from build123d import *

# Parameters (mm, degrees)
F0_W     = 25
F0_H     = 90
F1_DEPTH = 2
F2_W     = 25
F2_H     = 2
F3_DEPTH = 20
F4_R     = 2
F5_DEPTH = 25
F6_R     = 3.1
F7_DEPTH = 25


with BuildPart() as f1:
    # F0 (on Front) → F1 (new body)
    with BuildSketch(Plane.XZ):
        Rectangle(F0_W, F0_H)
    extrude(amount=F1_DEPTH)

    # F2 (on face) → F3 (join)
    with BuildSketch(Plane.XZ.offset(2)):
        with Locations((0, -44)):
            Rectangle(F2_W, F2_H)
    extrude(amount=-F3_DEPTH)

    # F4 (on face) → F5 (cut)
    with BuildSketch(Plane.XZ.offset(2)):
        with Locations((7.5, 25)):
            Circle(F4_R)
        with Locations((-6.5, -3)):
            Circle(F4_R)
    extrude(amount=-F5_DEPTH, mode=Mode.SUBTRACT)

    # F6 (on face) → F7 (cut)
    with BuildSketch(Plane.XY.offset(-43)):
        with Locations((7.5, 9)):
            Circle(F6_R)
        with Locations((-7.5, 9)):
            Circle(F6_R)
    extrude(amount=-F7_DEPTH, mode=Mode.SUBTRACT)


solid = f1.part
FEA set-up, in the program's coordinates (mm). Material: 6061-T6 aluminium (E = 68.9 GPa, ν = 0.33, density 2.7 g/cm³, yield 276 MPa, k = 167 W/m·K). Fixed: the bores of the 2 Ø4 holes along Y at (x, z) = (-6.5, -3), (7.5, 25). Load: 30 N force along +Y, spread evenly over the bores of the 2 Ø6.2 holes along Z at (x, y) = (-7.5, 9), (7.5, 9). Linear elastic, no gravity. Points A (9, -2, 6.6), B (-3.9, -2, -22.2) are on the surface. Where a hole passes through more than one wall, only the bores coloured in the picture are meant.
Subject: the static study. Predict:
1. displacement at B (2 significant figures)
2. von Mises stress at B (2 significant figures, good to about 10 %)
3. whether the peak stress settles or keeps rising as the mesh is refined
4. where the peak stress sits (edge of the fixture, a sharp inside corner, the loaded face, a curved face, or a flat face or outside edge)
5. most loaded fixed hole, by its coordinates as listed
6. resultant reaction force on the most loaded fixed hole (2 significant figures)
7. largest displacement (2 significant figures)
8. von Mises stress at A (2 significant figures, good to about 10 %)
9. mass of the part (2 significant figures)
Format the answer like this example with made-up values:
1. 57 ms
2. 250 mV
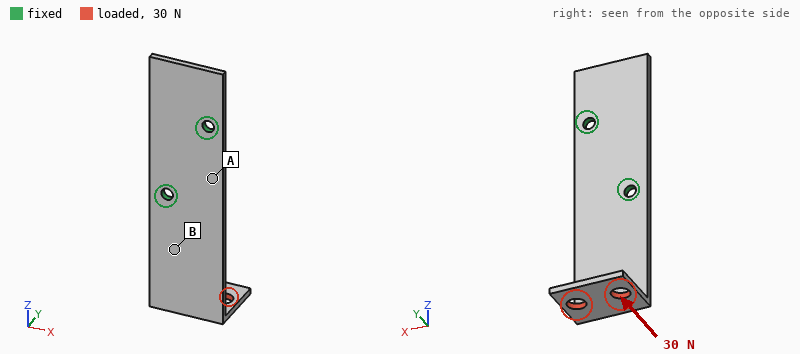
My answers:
1. 0.17 mm
2. 37 MPa
3. keeps rising
4. edge of the fixture
5. (-6.5, -3)
6. 43 N
7. 0.78 mm
8. 13 MPa
9. 14 g
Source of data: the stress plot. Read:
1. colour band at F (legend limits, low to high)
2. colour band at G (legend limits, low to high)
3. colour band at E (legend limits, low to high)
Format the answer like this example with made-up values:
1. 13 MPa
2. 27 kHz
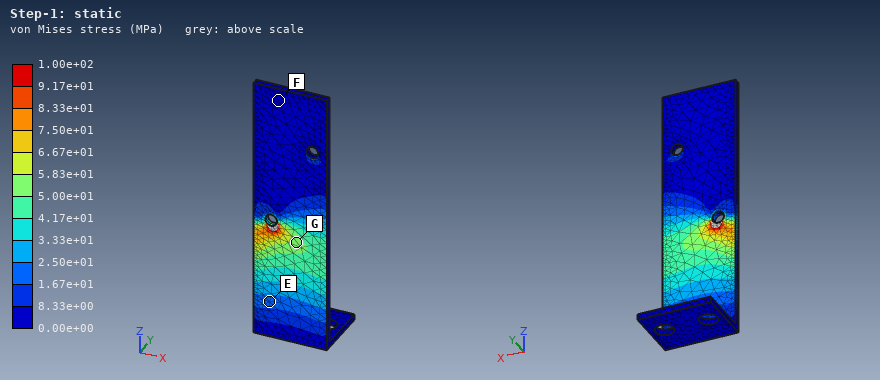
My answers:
1. 0.00e+00 to 8.33e+00 MPa
2. 5.00e+01 to 5.83e+01 MPa
3. 1.67e+01 to 2.50e+01 MPa
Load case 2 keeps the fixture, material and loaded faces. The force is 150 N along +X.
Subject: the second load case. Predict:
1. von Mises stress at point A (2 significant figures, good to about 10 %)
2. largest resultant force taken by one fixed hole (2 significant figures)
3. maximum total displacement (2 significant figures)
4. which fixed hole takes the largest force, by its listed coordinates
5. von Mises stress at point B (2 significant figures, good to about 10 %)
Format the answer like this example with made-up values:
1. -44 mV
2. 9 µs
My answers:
1. 42 MPa
2. 310 N
3. 0.90 mm
4. (-6.5, -3)
5. 76 MPa
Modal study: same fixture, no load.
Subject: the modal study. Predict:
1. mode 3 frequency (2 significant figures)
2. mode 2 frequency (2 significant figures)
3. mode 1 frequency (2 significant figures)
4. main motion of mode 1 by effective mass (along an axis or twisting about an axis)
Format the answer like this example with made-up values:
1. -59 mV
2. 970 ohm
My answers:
1. 2400 Hz
2. 1400 Hz
3. 560 Hz
4. along Y
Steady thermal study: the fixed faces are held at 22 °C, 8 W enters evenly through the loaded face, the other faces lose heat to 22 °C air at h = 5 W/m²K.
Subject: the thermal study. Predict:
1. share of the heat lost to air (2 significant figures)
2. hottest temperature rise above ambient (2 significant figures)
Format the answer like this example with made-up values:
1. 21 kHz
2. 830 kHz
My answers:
1. 6.1 %
2. 53 K
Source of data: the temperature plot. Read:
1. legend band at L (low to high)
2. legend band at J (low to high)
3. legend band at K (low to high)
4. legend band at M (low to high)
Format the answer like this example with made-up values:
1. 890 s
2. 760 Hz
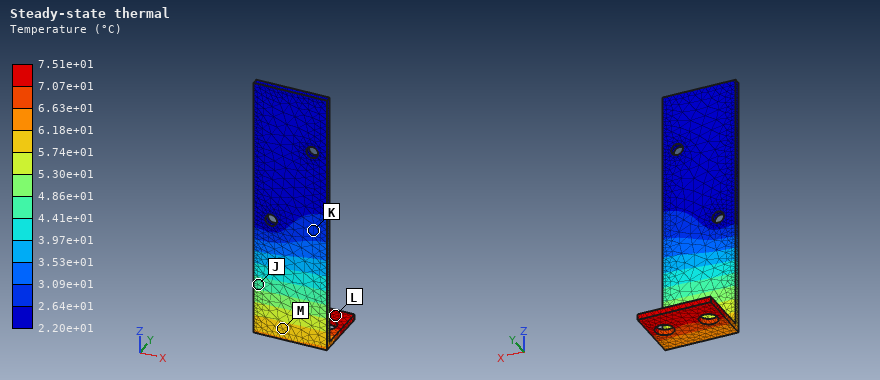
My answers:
1. 7.07e+01 to 7.51e+01 °C
2. 4.41e+01 to 4.86e+01 °C
3. 2.64e+01 to 3.09e+01 °C
4. 5.74e+01 to 6.18e+01 °C
